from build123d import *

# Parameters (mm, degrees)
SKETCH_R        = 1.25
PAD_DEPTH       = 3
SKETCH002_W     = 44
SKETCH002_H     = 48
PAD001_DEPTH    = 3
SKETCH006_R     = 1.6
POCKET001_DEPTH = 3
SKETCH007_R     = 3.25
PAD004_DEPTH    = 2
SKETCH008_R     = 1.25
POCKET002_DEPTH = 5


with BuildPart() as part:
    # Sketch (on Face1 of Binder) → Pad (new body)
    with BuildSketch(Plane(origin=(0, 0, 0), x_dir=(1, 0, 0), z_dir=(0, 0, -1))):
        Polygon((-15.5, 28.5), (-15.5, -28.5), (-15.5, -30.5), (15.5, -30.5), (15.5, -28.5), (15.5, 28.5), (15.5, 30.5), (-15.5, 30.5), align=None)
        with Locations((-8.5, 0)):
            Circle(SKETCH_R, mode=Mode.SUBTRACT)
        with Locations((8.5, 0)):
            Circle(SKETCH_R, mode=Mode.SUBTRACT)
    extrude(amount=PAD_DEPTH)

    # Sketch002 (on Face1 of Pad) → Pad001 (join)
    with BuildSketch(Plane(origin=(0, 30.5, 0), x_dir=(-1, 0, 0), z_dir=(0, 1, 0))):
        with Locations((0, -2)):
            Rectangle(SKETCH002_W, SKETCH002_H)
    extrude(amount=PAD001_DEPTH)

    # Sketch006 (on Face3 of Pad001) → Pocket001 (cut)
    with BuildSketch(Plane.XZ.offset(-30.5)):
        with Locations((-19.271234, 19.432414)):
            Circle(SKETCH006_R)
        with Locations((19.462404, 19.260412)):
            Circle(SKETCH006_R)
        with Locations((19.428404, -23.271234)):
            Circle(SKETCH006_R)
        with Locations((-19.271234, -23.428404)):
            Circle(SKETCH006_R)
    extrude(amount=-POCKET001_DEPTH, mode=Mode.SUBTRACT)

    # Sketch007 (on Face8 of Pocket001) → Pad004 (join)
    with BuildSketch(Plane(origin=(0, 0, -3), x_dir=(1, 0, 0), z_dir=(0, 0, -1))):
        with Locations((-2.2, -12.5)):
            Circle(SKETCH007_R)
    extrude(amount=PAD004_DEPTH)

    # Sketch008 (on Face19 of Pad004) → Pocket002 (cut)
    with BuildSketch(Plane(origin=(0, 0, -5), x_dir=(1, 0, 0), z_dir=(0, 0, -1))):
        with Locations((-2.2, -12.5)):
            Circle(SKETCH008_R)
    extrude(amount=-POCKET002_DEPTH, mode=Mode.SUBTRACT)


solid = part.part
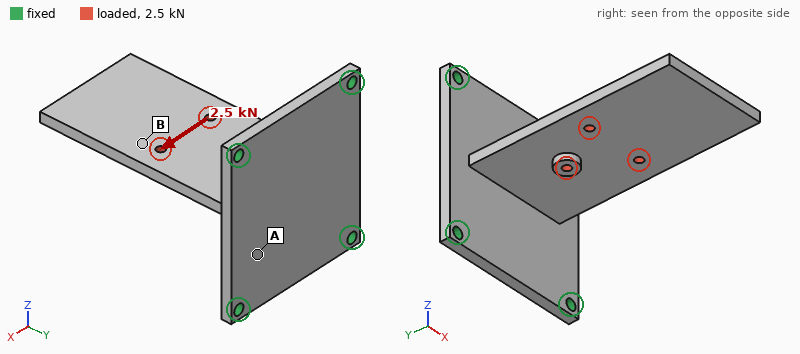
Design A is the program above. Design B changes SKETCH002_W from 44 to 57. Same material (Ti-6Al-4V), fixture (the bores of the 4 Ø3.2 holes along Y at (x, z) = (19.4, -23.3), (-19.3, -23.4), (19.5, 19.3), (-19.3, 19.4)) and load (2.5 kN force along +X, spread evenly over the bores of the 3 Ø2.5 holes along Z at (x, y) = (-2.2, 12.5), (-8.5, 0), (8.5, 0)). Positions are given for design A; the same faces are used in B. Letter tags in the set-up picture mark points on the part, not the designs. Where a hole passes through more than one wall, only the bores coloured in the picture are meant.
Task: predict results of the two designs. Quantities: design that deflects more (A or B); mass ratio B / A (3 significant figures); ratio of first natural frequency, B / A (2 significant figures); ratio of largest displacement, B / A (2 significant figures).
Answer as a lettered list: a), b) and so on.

a) A
b) 1.16
c) 1.0
d) 0.77
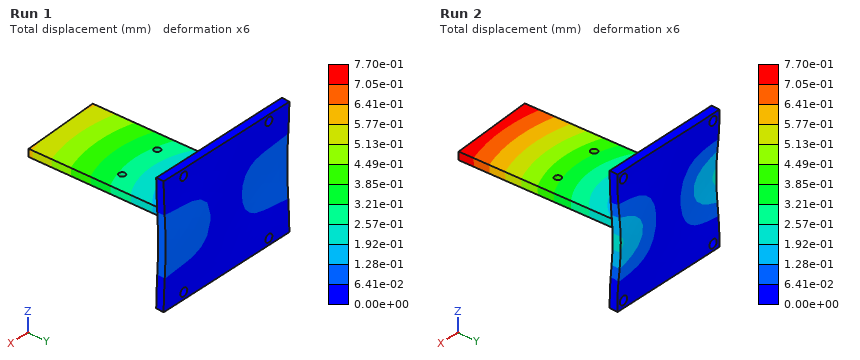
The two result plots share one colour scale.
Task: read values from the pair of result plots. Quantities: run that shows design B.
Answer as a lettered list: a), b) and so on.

a) Run 1
